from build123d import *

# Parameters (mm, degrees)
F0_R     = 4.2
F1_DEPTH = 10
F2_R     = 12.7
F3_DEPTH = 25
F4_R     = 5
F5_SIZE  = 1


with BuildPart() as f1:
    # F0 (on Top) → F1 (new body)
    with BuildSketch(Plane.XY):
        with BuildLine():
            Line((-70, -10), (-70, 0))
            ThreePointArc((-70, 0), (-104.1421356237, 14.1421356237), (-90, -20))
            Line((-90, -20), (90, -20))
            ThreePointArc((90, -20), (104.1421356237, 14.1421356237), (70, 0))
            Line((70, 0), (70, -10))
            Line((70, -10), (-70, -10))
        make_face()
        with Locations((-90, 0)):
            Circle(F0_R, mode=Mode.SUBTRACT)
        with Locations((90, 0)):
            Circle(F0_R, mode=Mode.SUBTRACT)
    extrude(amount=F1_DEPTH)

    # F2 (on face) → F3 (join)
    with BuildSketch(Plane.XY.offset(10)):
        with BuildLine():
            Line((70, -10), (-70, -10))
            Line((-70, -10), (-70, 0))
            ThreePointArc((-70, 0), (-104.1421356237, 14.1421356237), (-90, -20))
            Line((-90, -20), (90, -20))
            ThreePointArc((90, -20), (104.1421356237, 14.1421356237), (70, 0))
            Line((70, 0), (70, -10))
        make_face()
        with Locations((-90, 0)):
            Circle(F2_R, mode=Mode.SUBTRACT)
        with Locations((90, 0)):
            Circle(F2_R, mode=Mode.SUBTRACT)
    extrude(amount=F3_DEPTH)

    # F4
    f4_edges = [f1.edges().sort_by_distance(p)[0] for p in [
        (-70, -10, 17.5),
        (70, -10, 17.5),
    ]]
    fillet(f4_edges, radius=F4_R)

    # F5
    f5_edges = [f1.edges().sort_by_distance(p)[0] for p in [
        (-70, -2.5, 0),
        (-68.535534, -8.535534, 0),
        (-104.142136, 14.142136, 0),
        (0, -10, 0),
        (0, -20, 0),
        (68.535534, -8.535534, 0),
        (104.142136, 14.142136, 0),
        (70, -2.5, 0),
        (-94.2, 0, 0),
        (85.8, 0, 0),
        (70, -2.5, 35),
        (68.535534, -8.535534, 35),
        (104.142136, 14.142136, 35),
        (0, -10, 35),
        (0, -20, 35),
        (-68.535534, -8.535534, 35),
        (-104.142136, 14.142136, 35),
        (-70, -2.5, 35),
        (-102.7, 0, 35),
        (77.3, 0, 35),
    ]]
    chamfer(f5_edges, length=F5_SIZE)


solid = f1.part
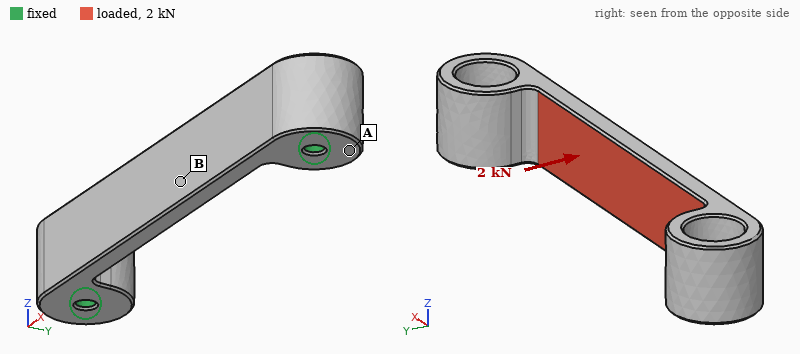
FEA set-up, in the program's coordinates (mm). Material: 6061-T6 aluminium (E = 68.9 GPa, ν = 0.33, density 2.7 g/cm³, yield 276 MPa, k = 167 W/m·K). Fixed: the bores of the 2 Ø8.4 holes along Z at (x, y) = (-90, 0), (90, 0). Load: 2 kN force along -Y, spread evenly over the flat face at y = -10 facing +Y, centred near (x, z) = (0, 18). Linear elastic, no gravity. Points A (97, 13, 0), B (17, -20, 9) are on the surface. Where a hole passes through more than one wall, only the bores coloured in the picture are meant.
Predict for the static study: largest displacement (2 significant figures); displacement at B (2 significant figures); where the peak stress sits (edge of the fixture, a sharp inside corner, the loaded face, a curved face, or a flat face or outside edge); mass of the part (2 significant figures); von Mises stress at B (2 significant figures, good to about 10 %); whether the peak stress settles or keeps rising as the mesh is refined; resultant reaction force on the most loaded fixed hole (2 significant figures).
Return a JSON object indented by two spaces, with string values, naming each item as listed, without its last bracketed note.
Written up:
{
  "largest displacement": "0.14 mm",
  "displacement at B": "0.11 mm",
  "where the peak stress sits": "edge of the fixture",
  "mass of the part": "310 g",
  "von Mises stress at B": "27 MPa",
  "whether the peak stress settles or keeps rising as the mesh is refined": "keeps rising",
  "resultant reaction force on the most loaded fixed hole": "1.6 kN"
}
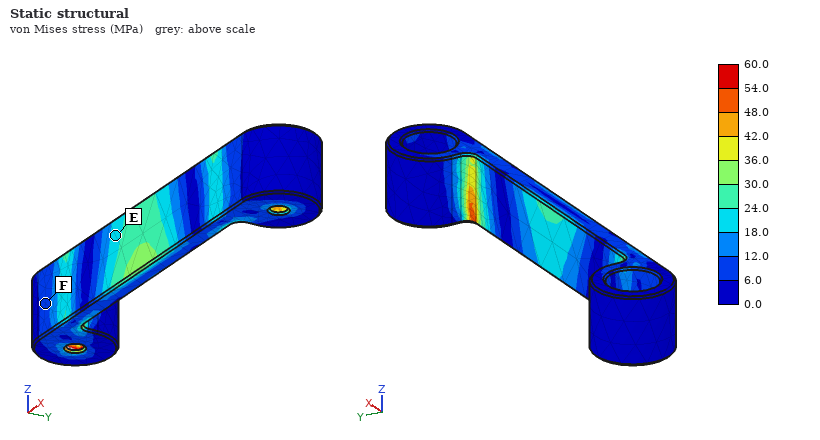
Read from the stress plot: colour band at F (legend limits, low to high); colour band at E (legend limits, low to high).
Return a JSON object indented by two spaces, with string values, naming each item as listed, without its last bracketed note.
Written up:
{
  "colour band at F": "6.0 to 12.0 MPa",
  "colour band at E": "18.0 to 24.0 MPa"
}
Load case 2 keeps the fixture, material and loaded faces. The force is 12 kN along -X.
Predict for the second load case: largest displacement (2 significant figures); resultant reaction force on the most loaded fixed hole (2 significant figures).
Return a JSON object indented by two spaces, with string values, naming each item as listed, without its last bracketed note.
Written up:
{
  "largest displacement": "66 µm",
  "resultant reaction force on the most loaded fixed hole": "6.0 kN"
}
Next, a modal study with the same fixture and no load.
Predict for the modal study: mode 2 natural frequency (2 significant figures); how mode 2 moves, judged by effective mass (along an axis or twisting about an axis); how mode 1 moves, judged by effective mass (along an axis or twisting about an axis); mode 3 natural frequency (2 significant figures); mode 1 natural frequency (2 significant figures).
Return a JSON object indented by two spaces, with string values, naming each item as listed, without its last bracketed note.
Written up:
{
  "mode 2 natural frequency": "3200 Hz",
  "how mode 2 moves, judged by effective mass": "along Z",
  "how mode 1 moves, judged by effective mass": "along Y",
  "mode 3 natural frequency": "4000 Hz",
  "mode 1 natural frequency": "2000 Hz"
}
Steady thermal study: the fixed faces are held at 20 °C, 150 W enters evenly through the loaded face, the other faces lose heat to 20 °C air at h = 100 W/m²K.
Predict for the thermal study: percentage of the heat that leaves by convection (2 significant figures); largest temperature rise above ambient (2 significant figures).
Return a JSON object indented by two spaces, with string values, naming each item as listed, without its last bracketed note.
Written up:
{
  "percentage of the heat that leaves by convection": "32 %",
  "largest temperature rise above ambient": "57 K"
}
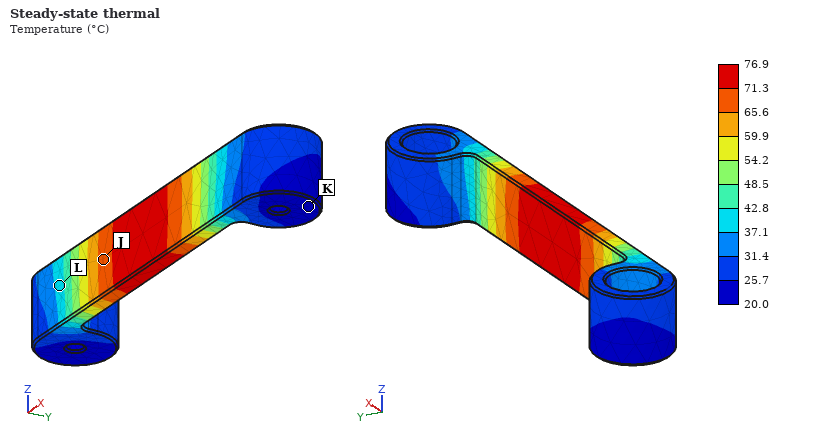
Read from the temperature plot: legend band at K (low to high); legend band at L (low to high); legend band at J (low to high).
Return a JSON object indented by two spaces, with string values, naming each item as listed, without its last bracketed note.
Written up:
{
  "legend band at K": "20.0 to 25.7 °C",
  "legend band at L": "37.1 to 42.8 °C",
  "legend band at J": "65.6 to 71.3 °C"
}
